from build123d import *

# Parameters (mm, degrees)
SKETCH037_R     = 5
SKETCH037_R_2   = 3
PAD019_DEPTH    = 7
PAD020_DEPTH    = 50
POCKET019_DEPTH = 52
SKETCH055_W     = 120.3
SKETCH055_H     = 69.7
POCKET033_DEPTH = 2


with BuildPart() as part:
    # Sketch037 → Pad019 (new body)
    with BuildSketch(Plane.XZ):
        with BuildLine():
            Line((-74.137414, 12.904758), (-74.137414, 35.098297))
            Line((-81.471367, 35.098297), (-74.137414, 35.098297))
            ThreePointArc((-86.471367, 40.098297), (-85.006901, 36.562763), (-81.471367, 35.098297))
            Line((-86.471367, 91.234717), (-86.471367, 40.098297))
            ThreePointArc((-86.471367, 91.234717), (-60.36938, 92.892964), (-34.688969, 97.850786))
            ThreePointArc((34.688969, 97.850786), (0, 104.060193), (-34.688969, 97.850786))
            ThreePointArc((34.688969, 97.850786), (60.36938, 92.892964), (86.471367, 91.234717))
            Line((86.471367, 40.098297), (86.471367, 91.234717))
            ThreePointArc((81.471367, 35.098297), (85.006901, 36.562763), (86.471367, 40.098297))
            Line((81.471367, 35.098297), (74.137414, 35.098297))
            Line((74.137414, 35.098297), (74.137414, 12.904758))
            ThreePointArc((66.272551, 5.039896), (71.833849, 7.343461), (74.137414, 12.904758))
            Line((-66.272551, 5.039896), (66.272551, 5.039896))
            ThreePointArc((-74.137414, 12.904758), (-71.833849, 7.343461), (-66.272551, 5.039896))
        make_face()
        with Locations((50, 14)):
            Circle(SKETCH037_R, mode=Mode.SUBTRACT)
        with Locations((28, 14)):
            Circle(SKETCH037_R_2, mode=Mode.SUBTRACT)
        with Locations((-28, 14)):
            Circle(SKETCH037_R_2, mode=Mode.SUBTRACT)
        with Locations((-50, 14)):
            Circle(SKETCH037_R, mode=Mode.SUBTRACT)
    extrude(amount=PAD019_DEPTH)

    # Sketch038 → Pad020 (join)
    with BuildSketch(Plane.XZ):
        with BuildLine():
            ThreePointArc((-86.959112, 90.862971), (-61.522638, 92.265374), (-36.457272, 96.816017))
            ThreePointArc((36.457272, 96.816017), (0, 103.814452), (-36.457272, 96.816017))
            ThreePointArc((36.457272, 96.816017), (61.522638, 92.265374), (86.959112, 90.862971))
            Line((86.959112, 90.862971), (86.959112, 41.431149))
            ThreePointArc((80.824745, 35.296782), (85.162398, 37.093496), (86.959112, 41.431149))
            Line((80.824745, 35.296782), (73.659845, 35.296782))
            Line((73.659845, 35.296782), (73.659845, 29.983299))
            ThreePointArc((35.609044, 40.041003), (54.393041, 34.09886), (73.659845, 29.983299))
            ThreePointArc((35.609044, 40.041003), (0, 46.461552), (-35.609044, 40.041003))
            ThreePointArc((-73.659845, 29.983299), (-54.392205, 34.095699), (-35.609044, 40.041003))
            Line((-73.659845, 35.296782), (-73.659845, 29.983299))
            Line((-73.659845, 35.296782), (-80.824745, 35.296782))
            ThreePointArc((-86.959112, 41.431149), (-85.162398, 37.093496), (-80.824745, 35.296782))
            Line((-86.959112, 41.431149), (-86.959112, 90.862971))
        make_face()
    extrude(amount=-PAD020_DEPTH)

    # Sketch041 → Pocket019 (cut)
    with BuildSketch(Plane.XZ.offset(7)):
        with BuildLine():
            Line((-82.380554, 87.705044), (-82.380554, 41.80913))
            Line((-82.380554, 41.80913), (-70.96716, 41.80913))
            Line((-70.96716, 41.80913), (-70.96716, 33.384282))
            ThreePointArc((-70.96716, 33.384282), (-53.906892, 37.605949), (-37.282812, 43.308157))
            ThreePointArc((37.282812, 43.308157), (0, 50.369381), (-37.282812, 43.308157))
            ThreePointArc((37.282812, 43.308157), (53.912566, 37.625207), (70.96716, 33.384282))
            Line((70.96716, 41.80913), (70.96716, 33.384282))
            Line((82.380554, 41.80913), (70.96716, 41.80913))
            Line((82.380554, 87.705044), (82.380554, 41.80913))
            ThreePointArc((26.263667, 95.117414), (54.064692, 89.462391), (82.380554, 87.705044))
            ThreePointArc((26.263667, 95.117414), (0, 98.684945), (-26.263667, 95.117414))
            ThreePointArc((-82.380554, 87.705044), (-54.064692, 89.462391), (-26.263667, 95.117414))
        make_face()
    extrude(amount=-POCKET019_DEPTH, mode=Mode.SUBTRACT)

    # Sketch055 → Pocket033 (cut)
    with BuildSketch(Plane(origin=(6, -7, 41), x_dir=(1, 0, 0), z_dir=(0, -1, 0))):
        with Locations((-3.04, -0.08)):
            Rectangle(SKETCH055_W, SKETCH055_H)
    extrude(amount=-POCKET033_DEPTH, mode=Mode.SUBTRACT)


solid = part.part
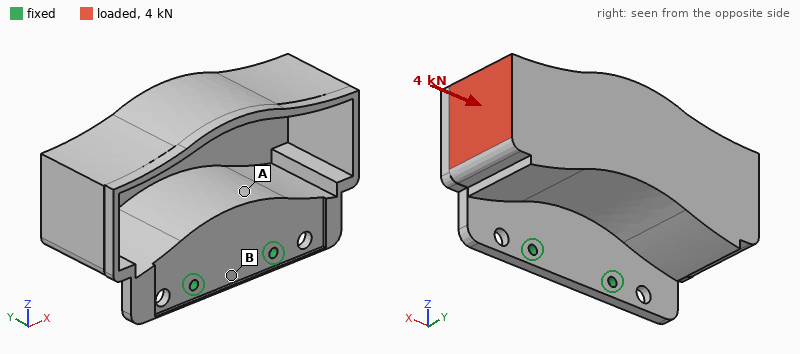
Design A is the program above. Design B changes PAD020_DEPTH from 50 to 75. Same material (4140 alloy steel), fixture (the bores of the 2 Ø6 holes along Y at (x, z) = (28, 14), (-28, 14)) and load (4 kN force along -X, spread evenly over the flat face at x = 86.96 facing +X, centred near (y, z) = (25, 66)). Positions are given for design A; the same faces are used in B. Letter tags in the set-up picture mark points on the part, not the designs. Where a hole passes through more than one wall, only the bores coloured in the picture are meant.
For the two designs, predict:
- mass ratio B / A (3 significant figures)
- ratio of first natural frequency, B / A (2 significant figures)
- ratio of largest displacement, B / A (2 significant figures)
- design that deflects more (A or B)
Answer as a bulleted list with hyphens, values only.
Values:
- 2.44
- 0.51
- 0.85
- A
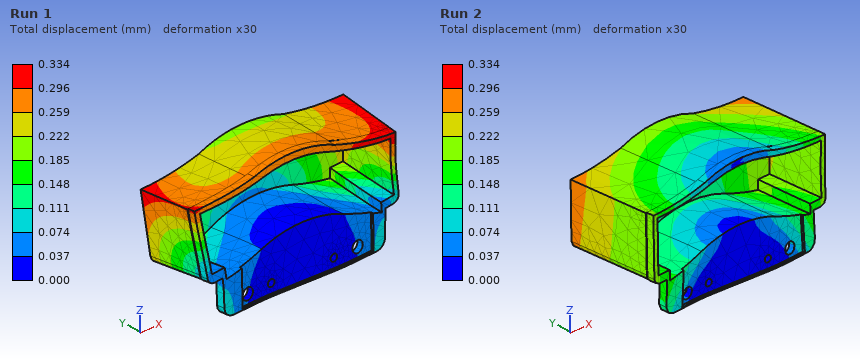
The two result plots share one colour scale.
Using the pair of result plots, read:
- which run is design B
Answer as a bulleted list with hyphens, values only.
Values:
- Run 2
